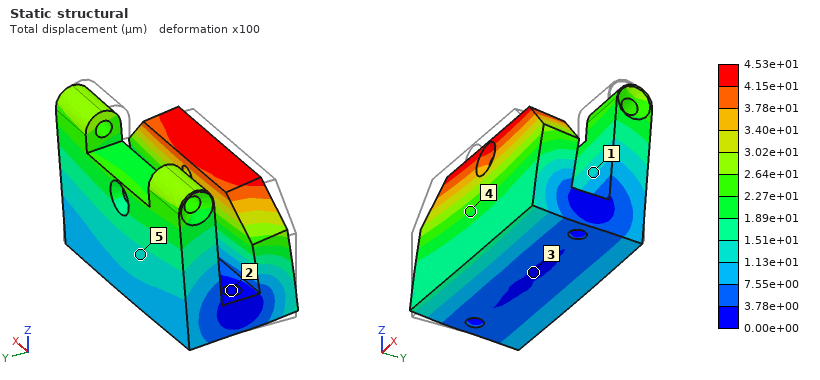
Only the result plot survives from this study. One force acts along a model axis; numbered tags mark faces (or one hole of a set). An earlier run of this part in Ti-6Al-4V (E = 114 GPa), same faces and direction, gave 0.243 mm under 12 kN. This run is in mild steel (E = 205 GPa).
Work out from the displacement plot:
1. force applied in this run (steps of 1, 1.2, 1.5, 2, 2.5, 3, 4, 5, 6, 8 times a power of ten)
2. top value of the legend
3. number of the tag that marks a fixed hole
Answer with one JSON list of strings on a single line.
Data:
["4 kN", "4.53e+01 µm", "2"]
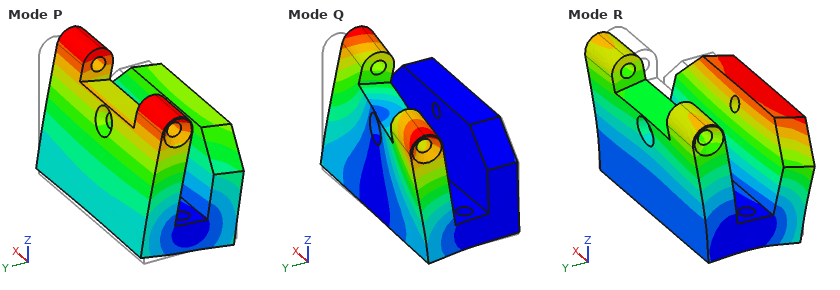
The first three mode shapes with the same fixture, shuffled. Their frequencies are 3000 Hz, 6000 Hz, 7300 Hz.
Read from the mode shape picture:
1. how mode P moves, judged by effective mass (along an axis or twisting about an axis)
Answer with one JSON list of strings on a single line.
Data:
["along Y"]
